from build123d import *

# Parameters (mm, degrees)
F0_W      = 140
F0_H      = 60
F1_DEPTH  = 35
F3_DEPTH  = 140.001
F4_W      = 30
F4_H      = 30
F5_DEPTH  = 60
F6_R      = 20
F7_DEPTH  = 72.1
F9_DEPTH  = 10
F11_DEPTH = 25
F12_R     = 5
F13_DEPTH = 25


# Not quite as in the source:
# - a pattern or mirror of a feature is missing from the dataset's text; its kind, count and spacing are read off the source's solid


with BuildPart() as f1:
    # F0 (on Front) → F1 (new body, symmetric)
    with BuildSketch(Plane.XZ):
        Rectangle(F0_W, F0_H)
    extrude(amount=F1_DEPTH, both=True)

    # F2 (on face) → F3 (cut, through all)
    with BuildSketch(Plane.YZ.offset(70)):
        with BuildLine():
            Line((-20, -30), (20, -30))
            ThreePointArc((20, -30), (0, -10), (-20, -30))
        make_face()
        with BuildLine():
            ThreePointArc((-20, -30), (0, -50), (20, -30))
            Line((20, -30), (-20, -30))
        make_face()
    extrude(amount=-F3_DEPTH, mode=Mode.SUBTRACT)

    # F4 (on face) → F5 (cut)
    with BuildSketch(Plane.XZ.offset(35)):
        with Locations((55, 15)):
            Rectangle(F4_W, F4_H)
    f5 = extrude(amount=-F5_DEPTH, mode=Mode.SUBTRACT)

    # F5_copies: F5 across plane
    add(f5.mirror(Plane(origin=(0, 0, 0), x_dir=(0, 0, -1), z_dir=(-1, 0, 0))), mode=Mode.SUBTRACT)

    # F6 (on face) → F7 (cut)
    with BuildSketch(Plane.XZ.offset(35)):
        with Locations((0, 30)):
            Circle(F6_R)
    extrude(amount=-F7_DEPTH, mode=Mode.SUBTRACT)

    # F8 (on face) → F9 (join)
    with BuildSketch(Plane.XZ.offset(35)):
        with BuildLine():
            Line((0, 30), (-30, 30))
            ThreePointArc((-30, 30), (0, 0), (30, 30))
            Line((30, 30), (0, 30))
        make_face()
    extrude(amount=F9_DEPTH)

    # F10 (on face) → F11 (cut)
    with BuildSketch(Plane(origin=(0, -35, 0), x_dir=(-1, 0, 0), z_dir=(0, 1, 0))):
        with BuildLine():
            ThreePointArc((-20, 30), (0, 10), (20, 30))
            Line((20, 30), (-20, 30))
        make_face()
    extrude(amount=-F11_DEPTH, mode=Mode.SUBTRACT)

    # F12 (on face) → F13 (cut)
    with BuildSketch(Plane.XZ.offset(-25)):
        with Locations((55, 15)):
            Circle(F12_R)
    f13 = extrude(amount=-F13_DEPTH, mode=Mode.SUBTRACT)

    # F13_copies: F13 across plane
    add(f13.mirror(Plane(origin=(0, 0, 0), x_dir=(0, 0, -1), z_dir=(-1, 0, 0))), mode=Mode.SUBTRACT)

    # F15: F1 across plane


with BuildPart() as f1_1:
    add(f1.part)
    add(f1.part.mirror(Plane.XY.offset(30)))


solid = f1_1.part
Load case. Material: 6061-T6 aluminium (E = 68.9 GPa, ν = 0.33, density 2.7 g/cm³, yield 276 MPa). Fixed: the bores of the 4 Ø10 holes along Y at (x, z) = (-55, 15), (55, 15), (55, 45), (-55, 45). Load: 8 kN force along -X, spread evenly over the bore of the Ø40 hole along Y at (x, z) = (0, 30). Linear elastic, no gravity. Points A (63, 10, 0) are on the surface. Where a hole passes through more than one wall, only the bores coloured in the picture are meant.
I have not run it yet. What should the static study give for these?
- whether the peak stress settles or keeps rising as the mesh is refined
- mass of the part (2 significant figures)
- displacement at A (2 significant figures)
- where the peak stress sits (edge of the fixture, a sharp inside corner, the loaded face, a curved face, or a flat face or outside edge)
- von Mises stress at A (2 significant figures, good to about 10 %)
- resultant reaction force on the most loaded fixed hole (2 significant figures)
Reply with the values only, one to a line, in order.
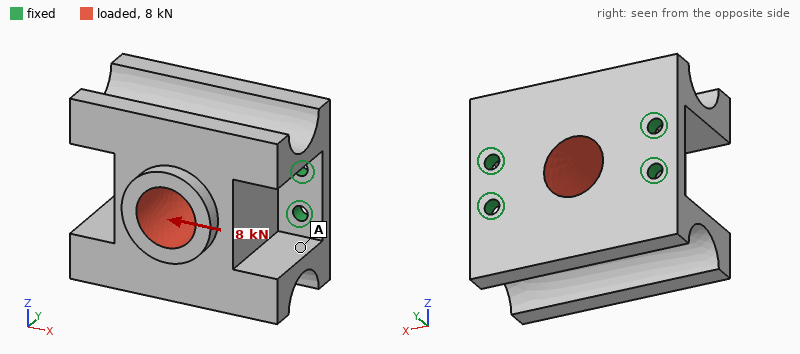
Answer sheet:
keeps rising
1.9 kg
6.3 µm
edge of the fixture
2.9 MPa
2.4 kN
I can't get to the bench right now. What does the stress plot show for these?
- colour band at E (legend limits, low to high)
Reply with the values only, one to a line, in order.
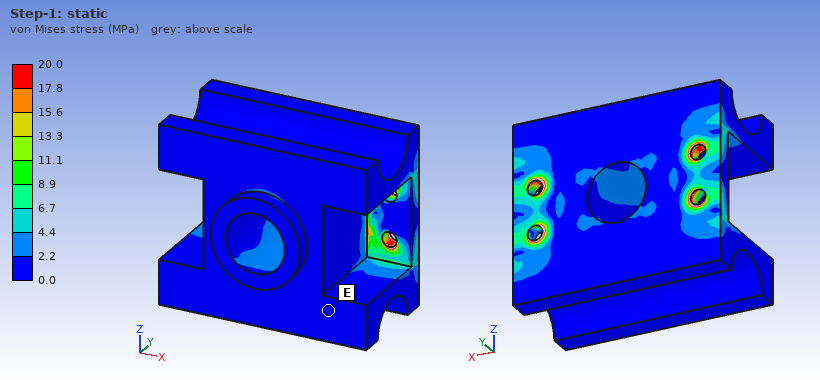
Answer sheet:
0.0 to 2.2 MPa
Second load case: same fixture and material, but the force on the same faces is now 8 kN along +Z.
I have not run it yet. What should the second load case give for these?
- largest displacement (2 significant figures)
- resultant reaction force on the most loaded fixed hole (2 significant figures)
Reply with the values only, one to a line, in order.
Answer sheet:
57 µm
3.7 kN
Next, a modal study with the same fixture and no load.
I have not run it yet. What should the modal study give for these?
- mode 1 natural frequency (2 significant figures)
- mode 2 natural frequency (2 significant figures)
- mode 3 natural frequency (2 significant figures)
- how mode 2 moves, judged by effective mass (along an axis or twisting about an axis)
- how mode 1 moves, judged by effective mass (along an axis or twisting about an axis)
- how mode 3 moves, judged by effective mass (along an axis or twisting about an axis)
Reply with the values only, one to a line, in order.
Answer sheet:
1500 Hz
3700 Hz
3900 Hz
along X
along Z
along Y
